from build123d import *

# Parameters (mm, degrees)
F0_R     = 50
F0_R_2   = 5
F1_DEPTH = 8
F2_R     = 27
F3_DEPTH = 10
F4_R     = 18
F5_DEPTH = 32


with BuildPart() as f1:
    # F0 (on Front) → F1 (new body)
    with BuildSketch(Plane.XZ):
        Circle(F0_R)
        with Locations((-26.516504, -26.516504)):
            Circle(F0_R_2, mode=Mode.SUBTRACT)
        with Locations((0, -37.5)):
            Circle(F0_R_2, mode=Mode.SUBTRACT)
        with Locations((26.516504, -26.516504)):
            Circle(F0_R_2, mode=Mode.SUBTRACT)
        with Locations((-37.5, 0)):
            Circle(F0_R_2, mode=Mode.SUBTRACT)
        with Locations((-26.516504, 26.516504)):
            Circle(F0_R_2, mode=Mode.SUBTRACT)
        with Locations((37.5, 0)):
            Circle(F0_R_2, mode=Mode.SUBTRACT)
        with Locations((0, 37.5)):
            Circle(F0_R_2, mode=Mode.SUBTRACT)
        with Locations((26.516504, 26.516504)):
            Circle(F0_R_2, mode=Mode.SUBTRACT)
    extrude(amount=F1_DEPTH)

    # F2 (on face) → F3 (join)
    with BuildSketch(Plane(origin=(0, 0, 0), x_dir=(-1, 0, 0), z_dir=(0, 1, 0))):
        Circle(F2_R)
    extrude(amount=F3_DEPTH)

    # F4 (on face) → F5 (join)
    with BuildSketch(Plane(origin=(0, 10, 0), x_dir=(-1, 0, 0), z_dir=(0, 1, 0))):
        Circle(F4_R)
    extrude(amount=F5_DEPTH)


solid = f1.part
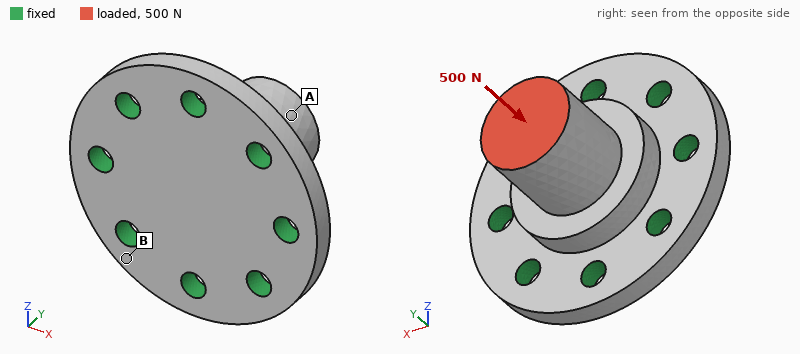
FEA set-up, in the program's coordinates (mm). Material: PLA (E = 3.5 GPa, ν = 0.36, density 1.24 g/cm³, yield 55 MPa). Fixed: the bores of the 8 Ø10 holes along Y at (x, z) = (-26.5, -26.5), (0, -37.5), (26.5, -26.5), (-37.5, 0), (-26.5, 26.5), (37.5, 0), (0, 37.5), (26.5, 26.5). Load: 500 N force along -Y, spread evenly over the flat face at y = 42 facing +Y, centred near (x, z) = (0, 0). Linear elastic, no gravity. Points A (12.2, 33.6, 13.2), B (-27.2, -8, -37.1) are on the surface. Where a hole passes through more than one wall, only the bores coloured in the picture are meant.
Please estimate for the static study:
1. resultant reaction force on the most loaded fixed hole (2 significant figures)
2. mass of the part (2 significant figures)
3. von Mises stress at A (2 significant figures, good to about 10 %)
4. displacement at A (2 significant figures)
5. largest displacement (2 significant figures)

78 N
140 g
0.48 MPa
12 µm
13 µm
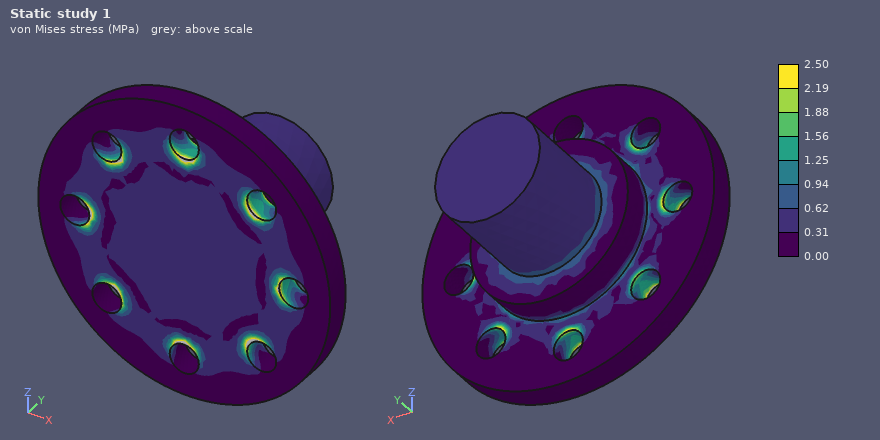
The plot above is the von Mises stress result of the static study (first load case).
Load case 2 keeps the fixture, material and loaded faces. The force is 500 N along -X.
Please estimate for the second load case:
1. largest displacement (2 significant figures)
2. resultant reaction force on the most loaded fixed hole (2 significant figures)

82 µm
230 N
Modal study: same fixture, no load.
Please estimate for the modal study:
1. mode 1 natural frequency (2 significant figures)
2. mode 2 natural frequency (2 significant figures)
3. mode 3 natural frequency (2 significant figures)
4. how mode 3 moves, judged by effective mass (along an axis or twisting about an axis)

3100 Hz
3100 Hz
4200 Hz
along Y
